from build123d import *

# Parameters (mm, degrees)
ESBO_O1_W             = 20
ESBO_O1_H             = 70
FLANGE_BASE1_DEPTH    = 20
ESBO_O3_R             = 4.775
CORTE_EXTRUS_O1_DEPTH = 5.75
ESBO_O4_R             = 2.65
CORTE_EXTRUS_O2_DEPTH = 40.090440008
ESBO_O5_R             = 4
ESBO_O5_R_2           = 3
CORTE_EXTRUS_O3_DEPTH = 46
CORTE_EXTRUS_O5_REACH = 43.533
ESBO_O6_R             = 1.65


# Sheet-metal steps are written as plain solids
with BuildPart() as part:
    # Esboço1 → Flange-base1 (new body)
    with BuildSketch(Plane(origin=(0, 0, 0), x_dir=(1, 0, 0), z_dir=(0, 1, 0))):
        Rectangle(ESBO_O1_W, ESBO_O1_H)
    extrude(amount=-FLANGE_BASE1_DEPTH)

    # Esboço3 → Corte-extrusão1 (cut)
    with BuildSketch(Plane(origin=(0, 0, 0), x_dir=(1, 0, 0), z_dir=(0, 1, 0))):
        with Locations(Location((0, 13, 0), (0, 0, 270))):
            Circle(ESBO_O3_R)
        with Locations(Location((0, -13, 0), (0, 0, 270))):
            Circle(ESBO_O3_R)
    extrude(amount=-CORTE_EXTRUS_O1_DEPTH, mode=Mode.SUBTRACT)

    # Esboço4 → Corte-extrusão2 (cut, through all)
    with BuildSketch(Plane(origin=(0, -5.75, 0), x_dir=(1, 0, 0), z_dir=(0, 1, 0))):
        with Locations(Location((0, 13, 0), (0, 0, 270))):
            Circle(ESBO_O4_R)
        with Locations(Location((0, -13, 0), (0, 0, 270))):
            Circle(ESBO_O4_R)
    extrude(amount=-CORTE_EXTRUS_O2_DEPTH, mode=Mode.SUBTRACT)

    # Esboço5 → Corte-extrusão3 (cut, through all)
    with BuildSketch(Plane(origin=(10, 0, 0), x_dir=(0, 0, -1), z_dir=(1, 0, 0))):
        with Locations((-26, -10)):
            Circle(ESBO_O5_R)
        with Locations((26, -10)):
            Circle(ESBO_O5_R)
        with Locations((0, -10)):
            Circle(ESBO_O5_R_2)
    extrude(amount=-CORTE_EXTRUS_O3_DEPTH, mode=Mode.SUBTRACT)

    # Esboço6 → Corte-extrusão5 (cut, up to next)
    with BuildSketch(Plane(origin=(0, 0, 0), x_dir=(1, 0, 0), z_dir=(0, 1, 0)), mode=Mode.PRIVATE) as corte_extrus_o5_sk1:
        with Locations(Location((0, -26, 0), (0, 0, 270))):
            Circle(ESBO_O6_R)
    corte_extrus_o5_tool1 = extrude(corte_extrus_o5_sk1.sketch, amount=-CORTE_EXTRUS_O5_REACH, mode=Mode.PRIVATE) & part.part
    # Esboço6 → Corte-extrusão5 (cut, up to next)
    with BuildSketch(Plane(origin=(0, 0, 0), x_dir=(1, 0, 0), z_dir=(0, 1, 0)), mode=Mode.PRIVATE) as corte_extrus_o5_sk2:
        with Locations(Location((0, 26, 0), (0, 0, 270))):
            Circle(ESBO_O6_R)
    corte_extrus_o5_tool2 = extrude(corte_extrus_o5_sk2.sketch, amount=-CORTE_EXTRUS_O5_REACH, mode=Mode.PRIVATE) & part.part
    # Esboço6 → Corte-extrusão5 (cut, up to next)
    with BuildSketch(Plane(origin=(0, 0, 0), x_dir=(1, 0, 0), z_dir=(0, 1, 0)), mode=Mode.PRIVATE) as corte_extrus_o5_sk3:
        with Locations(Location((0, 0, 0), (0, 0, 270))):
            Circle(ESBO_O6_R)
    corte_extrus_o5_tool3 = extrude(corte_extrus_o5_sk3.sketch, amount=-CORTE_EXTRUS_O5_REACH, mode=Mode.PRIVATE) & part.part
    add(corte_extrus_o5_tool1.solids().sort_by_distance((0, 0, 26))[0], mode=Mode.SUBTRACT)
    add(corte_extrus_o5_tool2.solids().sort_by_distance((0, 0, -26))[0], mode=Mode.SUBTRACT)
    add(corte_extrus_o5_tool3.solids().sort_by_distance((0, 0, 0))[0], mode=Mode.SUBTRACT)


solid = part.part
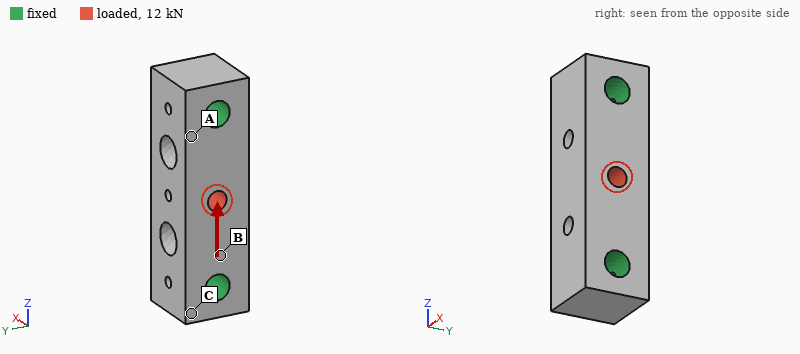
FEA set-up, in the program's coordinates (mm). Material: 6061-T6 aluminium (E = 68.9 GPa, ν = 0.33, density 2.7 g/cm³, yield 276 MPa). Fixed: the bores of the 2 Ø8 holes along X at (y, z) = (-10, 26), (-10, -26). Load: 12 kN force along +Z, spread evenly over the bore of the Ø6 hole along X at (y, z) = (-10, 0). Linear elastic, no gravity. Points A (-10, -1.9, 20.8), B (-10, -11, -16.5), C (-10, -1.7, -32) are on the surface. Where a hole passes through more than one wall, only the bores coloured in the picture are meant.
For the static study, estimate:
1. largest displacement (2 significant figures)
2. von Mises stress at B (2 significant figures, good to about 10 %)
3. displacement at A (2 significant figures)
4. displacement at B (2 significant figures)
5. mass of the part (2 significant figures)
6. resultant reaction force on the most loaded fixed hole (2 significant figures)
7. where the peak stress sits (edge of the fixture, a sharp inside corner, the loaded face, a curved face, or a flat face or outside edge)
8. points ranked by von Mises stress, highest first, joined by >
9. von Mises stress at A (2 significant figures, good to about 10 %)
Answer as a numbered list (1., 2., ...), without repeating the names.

1. 8.2 µm
2. 25 MPa
3. 2.1 µm
4. 2.6 µm
5. 64 g
6. 6.0 kN
7. the loaded face
8. B > A > C
9. 14 MPa
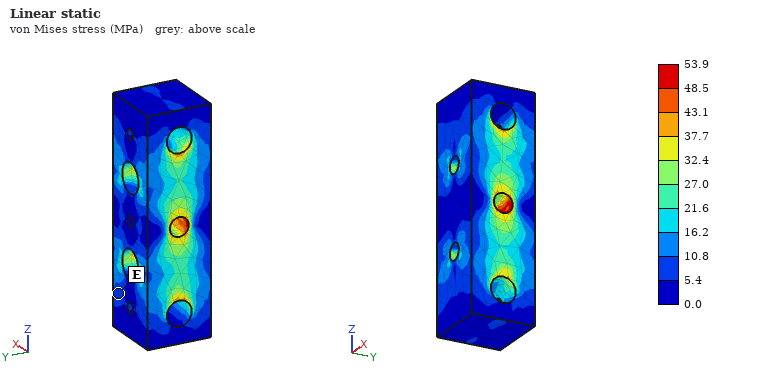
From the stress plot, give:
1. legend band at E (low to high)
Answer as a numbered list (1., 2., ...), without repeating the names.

1. 5.4 to 10.8 MPa
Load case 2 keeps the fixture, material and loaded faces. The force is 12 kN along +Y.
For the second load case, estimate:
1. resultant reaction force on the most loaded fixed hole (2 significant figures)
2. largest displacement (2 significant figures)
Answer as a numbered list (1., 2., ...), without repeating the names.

1. 6.0 kN
2. 32 µm
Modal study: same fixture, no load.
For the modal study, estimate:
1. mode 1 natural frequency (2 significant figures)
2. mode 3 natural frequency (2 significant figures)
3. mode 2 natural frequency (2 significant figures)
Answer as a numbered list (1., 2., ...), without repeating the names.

1. 22 kHz
2. 27 kHz
3. 22 kHz
